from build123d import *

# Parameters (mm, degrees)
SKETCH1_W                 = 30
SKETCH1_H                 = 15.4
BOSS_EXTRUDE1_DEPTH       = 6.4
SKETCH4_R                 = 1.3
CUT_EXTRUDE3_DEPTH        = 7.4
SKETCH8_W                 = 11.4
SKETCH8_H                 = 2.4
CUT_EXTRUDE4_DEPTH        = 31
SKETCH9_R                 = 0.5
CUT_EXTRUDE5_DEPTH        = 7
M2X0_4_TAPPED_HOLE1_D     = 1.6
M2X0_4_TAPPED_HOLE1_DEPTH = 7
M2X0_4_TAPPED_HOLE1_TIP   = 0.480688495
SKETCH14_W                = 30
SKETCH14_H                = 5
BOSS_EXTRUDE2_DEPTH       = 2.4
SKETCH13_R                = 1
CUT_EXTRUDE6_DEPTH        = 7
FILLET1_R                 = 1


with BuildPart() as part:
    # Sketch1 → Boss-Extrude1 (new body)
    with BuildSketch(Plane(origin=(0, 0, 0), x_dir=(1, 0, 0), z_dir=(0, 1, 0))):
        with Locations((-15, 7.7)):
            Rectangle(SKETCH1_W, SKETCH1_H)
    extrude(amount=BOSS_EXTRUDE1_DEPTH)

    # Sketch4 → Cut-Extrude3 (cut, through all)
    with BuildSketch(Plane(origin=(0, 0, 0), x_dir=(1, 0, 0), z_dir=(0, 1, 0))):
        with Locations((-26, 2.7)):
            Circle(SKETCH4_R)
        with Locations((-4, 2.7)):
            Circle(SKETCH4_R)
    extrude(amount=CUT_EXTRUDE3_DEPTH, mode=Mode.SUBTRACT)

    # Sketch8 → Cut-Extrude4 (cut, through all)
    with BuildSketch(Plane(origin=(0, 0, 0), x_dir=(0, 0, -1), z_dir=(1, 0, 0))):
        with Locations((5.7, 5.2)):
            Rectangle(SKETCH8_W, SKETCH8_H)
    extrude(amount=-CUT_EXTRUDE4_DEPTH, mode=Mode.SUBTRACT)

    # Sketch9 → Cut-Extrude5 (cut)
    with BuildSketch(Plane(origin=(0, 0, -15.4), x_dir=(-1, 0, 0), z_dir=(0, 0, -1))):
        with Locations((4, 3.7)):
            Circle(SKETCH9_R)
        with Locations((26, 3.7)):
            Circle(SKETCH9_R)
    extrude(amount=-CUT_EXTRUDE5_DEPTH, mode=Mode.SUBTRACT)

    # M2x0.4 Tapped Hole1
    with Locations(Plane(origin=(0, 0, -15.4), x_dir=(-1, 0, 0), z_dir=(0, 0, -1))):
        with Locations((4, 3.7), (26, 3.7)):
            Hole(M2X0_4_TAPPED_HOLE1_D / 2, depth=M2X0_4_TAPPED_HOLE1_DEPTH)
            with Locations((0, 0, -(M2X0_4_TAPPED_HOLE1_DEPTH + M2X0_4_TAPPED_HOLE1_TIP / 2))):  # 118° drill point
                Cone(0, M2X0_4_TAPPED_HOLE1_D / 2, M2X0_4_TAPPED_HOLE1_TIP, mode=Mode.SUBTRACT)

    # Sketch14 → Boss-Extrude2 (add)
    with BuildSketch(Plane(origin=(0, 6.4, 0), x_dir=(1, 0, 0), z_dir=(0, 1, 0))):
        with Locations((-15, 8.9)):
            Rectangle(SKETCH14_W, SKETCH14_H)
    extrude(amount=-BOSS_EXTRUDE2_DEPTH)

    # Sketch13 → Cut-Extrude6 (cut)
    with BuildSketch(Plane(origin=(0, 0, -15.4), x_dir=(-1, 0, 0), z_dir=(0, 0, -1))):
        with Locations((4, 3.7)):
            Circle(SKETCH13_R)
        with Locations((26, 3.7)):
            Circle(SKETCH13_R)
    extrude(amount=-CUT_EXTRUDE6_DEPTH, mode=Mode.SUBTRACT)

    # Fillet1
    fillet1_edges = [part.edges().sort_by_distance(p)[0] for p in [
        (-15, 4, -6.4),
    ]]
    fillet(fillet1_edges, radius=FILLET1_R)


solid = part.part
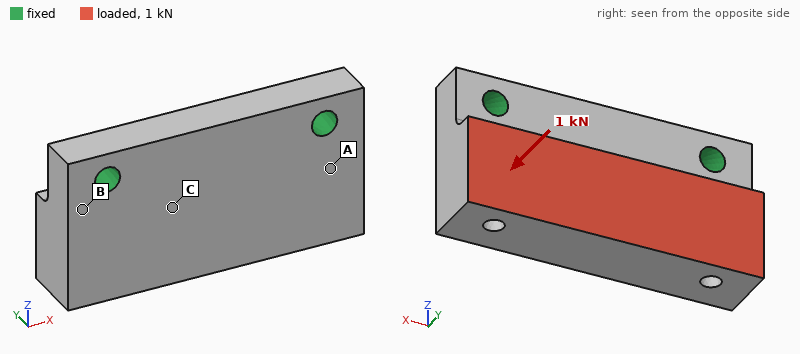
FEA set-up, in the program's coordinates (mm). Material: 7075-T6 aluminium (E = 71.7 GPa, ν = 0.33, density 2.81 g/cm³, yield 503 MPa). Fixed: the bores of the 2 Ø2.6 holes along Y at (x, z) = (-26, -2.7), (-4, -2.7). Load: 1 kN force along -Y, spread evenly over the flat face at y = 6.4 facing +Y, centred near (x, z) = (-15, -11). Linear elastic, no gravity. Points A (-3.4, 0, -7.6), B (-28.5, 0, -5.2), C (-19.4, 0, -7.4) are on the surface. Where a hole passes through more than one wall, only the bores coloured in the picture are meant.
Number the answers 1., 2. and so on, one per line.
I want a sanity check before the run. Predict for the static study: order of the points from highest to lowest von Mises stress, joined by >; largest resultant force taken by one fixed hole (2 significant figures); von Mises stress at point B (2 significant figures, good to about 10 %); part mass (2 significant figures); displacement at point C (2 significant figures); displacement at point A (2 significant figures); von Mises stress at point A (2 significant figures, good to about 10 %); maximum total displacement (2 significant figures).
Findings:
1. B > A > C
2. 500 N
3. 85 MPa
4. 6.8 g
5. 18 µm
6. 14 µm
7. 49 MPa
8. 51 µm
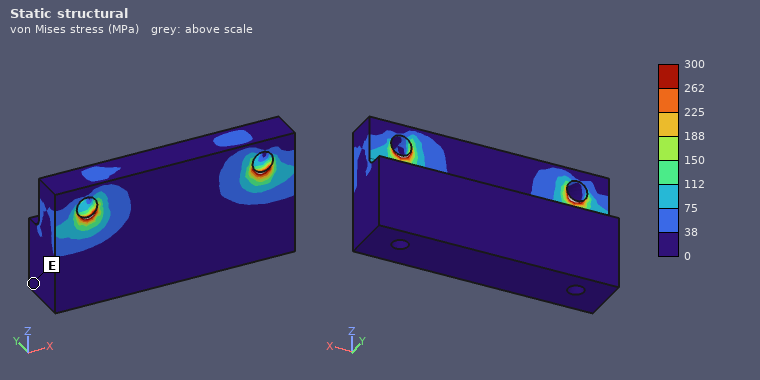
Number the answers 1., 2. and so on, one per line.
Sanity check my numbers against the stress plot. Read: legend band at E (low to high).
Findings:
1. 0 to 38 MPa
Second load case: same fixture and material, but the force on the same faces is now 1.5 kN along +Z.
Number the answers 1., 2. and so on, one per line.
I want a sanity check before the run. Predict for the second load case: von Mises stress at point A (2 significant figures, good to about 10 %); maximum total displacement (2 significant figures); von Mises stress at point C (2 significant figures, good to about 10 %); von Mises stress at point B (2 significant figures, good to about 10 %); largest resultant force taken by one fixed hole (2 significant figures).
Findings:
1. 49 MPa
2. 50 µm
3. 30 MPa
4. 80 MPa
5. 770 N
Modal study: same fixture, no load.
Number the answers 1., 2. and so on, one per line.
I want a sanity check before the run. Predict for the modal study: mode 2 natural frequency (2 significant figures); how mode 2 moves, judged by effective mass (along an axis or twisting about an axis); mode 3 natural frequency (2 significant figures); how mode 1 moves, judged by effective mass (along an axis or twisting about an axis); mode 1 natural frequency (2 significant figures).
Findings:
1. 26 kHz
2. twisting about Z
3. 38 kHz
4. along Y
5. 12 kHz
